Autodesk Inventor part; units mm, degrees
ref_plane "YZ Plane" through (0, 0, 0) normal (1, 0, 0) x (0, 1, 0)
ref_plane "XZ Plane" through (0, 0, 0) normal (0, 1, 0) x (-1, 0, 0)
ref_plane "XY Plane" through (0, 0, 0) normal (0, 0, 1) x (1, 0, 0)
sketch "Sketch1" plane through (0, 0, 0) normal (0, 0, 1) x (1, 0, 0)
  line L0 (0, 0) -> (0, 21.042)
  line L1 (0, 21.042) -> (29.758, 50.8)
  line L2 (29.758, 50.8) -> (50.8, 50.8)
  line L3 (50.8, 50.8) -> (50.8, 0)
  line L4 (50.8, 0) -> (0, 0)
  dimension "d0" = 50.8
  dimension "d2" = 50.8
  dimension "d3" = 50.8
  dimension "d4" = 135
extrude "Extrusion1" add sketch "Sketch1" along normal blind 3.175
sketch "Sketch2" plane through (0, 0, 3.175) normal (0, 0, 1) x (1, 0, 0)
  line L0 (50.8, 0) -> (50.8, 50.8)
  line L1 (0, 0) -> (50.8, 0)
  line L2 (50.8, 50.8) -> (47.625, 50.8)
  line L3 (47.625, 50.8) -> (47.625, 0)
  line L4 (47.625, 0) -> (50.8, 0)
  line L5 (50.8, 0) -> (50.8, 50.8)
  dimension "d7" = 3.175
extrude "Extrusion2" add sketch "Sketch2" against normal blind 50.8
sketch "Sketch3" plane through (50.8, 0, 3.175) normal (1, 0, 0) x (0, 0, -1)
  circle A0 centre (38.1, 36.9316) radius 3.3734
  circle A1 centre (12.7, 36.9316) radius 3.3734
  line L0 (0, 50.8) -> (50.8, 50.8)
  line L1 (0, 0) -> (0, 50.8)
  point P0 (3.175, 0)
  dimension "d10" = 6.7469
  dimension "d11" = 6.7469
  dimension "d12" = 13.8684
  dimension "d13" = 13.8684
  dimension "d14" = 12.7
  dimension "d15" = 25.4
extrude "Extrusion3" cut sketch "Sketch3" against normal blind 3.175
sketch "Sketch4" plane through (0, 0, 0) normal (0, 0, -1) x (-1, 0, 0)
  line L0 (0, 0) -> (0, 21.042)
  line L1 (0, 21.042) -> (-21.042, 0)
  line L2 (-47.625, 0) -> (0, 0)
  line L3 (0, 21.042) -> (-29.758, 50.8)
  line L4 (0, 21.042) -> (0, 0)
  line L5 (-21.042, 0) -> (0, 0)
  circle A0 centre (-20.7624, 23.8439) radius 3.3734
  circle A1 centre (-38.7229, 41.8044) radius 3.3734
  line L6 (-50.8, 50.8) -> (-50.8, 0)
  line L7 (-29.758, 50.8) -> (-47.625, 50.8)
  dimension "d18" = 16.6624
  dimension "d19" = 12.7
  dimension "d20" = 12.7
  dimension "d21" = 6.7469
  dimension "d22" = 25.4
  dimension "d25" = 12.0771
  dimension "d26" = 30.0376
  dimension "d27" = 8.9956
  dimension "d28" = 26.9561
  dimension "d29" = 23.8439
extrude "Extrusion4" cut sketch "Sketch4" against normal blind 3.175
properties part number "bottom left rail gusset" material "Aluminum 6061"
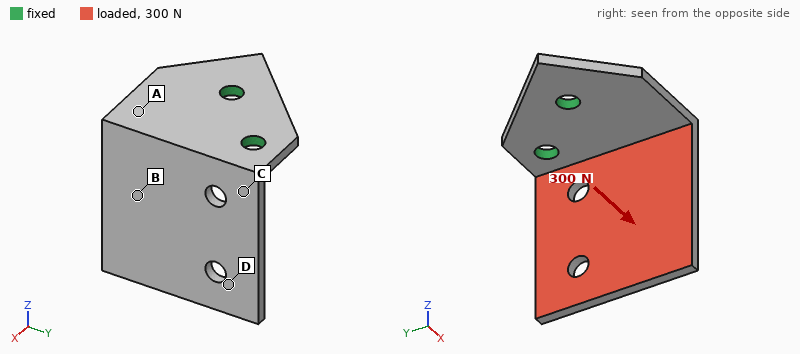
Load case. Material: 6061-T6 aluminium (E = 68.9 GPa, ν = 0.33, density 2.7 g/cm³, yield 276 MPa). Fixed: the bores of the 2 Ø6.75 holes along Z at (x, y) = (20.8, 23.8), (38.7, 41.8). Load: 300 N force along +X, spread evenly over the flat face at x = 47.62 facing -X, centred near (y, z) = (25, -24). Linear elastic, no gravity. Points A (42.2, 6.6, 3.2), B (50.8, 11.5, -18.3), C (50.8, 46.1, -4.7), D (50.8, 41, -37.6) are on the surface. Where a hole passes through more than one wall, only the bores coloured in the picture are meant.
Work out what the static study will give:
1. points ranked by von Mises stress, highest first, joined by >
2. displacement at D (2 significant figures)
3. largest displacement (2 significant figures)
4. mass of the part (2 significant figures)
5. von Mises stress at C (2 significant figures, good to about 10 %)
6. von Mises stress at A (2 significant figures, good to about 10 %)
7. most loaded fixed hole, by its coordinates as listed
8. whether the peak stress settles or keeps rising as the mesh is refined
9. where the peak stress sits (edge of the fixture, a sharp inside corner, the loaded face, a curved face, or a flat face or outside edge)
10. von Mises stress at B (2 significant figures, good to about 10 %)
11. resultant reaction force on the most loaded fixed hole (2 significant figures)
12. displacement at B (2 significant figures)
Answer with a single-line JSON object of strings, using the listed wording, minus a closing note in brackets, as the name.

{"points ranked by von Mises stress, highest first, joined by >": "C > A > B > D", "displacement at D": "0.71 mm", "largest displacement": "1.0 mm", "mass of the part": "36 g", "von Mises stress at C": "81 MPa", "von Mises stress at A": "58 MPa", "most loaded fixed hole, by its coordinates as listed": "(20.8, 23.8)", "whether the peak stress settles or keeps rising as the mesh is refined": "keeps rising", "where the peak stress sits": "edge of the fixture", "von Mises stress at B": "28 MPa", "resultant reaction force on the most loaded fixed hole": "260 N", "displacement at B": "0.36 mm"}
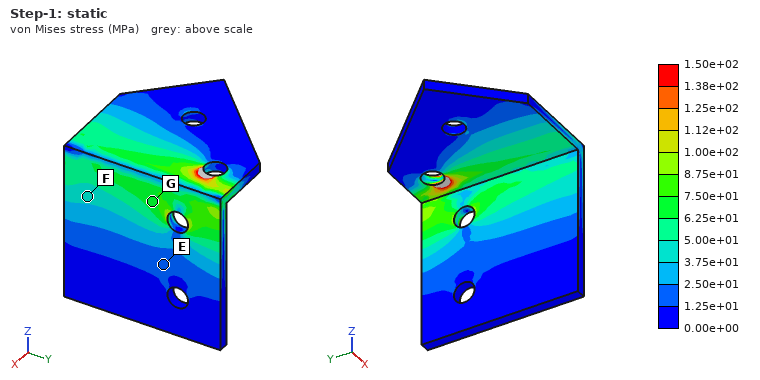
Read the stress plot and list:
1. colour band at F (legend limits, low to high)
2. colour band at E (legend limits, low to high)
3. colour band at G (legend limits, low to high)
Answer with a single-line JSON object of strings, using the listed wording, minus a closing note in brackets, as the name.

{"colour band at F": "3.75e+01 to 5.00e+01 MPa", "colour band at E": "1.25e+01 to 2.50e+01 MPa", "colour band at G": "6.25e+01 to 7.50e+01 MPa"}
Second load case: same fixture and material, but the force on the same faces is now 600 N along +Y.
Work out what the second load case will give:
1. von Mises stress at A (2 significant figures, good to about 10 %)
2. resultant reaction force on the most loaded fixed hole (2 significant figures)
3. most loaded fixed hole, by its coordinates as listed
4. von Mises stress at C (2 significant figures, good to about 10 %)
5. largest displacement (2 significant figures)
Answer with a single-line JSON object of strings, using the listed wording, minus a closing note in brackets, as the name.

{"von Mises stress at A": "24 MPa", "resultant reaction force on the most loaded fixed hole": "640 N", "most loaded fixed hole, by its coordinates as listed": "(38.7, 41.8)", "von Mises stress at C": "41 MPa", "largest displacement": "0.71 mm"}
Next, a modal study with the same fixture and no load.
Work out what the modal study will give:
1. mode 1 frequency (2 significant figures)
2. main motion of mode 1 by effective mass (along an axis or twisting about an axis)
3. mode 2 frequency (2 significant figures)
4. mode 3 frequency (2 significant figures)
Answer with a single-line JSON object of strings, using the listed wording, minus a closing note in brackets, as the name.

{"mode 1 frequency": "750 Hz", "main motion of mode 1 by effective mass": "along X", "mode 2 frequency": "1400 Hz", "mode 3 frequency": "2300 Hz"}
